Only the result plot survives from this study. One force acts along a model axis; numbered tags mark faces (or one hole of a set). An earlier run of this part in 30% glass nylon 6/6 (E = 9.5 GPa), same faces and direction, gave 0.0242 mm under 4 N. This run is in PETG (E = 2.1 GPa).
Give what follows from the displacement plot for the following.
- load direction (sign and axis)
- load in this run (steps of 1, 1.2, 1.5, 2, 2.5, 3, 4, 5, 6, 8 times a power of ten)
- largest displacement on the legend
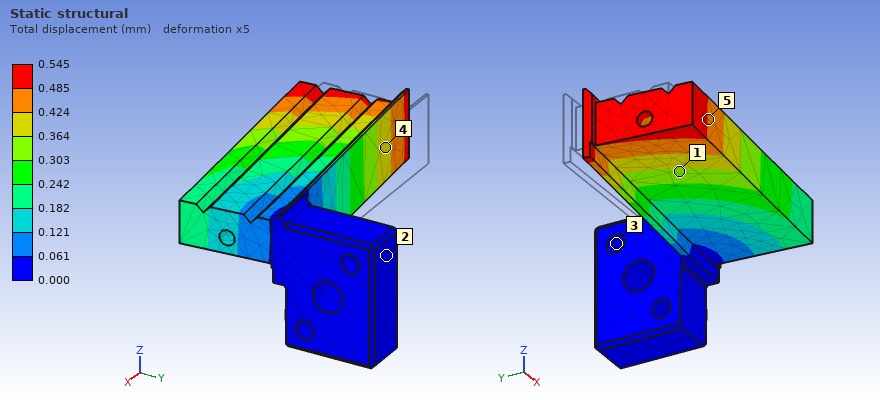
-Y
20 N
0.545 mm
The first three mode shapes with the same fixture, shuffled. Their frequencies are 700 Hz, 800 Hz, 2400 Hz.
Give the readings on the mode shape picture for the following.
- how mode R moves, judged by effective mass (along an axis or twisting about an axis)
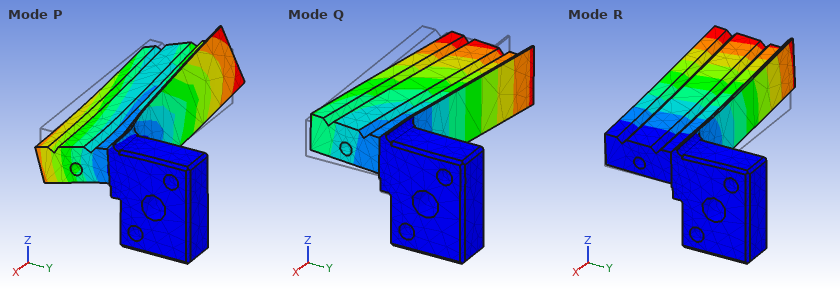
along Z
